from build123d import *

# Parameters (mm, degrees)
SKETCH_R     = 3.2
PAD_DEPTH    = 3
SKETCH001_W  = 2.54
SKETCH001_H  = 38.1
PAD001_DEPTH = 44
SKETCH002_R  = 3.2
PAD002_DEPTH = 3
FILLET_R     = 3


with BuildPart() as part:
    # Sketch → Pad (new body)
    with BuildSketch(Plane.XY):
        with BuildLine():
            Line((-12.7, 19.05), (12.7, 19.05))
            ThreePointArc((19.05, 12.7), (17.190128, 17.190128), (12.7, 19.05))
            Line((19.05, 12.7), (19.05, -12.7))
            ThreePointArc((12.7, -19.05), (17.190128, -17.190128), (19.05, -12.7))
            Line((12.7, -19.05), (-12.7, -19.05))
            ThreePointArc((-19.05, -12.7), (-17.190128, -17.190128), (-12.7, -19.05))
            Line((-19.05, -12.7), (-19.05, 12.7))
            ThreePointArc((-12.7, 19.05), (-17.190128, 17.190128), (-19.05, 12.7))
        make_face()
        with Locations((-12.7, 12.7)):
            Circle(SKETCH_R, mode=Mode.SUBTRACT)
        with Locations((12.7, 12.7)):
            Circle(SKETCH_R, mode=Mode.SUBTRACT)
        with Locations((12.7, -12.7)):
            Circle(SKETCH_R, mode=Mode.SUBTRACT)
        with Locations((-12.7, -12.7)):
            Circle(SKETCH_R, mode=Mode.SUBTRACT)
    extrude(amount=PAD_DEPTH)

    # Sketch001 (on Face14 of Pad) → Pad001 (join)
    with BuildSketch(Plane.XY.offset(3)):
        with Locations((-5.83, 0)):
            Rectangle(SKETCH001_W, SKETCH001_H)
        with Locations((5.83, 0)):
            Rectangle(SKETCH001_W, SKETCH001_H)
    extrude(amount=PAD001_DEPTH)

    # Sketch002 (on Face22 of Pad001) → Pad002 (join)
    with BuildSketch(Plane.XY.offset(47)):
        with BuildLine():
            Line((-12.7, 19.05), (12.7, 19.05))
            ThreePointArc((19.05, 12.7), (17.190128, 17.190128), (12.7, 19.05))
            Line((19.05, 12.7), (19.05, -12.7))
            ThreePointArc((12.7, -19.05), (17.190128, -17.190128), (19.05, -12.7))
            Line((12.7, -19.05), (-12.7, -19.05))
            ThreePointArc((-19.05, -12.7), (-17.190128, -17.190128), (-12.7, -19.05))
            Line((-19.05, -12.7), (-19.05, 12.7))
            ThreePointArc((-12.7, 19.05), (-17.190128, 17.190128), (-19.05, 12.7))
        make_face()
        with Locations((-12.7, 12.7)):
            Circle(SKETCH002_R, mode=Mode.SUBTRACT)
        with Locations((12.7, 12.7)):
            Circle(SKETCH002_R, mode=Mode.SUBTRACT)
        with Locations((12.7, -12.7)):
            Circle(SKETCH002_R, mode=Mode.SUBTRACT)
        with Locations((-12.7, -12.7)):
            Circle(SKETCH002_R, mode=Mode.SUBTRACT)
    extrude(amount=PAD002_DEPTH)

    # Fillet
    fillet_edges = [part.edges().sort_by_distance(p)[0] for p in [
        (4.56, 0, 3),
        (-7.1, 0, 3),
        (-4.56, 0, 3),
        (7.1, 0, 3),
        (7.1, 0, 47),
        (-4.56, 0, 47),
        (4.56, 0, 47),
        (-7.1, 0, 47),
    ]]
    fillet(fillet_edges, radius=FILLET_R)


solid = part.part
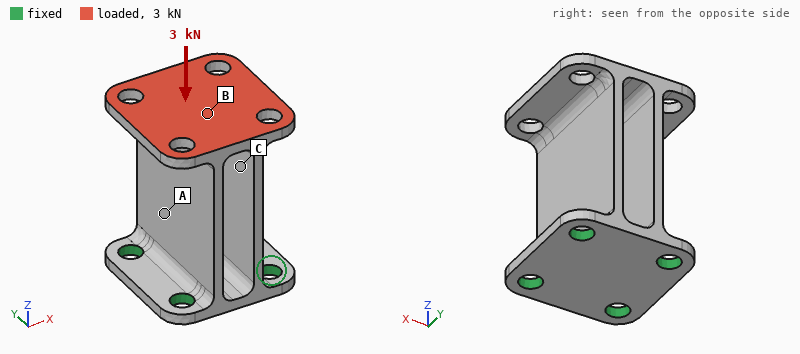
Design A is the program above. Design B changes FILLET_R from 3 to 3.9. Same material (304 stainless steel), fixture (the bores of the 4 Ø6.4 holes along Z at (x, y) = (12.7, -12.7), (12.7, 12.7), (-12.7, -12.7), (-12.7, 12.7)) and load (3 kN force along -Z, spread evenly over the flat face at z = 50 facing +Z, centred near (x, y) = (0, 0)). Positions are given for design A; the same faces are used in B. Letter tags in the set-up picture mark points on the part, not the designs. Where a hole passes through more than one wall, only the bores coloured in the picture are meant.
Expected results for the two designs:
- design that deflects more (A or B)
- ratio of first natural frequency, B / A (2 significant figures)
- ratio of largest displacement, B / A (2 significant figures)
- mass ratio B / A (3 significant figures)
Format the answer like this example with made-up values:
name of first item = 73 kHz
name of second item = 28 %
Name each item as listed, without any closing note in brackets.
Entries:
design that deflects more = A
ratio of first natural frequency, B / A = 1.0
ratio of largest displacement, B / A = 0.89
mass ratio B / A = 1.02
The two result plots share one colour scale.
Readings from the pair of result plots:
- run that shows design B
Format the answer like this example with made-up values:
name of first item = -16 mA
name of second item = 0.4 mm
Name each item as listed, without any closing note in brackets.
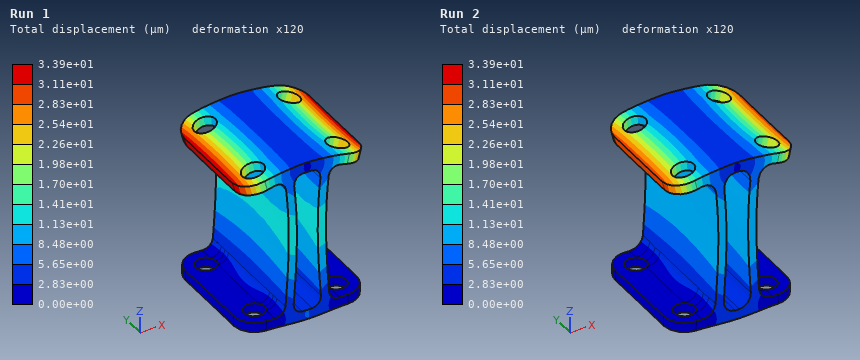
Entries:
run that shows design B = Run 2
